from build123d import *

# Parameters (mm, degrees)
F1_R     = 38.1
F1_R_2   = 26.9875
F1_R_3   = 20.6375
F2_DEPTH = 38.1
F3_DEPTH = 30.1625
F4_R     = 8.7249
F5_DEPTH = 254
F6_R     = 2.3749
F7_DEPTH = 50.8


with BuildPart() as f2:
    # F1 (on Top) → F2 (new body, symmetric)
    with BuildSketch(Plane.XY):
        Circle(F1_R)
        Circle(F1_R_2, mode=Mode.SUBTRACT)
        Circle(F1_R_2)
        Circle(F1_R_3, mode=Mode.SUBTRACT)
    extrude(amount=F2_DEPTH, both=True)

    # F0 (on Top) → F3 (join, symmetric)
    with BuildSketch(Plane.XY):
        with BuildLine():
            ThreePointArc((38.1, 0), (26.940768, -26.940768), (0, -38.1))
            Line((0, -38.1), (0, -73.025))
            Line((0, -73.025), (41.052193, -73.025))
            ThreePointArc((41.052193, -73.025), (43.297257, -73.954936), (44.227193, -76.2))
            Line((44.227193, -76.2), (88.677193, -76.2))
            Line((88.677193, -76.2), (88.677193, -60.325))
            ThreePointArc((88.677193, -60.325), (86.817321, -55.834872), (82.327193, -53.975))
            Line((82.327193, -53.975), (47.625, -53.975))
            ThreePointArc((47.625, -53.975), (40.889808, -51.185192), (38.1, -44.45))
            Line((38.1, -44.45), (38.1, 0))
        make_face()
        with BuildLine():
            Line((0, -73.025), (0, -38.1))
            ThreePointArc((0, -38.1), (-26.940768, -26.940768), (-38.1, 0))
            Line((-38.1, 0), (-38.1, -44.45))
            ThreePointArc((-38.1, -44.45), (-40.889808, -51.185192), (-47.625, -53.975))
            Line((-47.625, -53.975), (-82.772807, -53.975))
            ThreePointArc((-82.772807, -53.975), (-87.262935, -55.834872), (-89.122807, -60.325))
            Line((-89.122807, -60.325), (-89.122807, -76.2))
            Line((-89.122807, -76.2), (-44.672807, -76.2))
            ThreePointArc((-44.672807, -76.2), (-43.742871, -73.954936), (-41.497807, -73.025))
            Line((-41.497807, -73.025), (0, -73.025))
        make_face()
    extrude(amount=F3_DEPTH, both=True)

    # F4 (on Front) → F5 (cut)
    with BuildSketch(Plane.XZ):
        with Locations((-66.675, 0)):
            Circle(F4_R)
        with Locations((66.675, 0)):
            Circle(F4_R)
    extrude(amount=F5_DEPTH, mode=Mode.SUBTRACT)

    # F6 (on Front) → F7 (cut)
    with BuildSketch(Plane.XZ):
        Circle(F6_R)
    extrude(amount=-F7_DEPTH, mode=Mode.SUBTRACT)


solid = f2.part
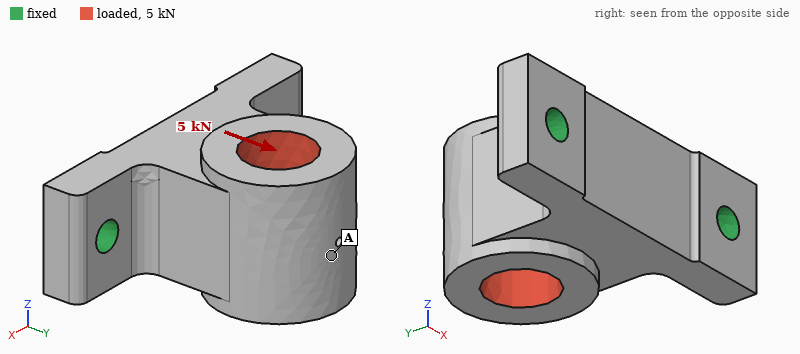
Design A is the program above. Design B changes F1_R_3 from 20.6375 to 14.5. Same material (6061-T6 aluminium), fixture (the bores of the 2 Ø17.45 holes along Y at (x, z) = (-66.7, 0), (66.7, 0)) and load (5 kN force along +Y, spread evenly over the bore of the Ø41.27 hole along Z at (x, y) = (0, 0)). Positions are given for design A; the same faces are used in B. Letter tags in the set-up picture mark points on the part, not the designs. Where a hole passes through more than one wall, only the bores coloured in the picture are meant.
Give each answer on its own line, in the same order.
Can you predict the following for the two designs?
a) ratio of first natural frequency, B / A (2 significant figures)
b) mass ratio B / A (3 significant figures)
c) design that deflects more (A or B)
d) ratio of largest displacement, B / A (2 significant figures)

0.93
1.09
A
0.91
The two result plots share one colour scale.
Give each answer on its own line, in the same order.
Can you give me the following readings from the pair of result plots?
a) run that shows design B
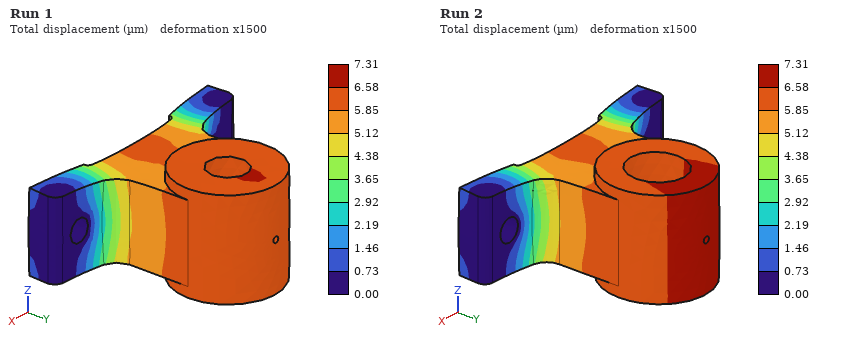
Run 1
